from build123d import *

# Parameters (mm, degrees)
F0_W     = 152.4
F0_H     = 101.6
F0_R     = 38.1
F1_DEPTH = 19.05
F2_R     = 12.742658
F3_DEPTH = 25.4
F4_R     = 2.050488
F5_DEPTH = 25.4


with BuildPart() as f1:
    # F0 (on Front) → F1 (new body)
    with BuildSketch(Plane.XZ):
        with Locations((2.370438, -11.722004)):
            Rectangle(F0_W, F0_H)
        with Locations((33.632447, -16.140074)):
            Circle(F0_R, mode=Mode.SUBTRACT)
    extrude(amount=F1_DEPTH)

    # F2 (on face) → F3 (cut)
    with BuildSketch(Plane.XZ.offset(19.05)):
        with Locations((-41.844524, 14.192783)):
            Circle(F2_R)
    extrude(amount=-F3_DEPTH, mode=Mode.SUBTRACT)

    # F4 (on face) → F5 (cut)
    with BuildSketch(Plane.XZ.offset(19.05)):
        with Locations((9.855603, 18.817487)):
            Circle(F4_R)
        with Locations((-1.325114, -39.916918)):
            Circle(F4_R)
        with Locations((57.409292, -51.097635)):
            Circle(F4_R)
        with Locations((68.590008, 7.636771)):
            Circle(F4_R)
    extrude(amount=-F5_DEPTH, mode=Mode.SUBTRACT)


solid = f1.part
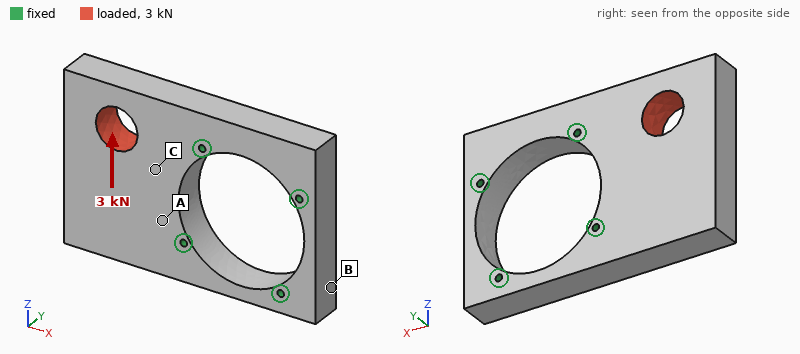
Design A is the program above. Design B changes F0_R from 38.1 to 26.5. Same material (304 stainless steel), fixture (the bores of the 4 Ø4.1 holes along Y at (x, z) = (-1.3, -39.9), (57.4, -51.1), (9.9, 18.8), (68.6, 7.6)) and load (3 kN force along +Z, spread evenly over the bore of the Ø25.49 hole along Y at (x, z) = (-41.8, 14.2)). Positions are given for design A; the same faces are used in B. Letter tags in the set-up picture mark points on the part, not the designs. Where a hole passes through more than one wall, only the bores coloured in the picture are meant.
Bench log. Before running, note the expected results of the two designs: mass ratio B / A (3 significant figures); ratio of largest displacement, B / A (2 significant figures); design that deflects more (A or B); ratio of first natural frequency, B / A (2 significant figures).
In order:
1.23
0.86
A
1.1
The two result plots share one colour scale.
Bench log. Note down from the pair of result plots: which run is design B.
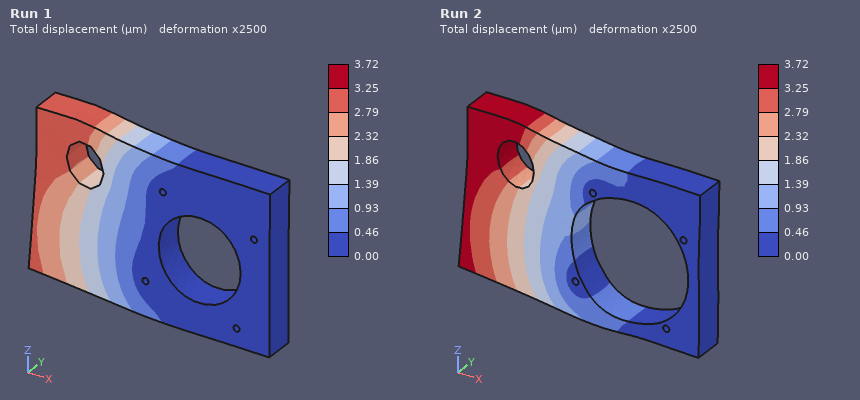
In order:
Run 1
